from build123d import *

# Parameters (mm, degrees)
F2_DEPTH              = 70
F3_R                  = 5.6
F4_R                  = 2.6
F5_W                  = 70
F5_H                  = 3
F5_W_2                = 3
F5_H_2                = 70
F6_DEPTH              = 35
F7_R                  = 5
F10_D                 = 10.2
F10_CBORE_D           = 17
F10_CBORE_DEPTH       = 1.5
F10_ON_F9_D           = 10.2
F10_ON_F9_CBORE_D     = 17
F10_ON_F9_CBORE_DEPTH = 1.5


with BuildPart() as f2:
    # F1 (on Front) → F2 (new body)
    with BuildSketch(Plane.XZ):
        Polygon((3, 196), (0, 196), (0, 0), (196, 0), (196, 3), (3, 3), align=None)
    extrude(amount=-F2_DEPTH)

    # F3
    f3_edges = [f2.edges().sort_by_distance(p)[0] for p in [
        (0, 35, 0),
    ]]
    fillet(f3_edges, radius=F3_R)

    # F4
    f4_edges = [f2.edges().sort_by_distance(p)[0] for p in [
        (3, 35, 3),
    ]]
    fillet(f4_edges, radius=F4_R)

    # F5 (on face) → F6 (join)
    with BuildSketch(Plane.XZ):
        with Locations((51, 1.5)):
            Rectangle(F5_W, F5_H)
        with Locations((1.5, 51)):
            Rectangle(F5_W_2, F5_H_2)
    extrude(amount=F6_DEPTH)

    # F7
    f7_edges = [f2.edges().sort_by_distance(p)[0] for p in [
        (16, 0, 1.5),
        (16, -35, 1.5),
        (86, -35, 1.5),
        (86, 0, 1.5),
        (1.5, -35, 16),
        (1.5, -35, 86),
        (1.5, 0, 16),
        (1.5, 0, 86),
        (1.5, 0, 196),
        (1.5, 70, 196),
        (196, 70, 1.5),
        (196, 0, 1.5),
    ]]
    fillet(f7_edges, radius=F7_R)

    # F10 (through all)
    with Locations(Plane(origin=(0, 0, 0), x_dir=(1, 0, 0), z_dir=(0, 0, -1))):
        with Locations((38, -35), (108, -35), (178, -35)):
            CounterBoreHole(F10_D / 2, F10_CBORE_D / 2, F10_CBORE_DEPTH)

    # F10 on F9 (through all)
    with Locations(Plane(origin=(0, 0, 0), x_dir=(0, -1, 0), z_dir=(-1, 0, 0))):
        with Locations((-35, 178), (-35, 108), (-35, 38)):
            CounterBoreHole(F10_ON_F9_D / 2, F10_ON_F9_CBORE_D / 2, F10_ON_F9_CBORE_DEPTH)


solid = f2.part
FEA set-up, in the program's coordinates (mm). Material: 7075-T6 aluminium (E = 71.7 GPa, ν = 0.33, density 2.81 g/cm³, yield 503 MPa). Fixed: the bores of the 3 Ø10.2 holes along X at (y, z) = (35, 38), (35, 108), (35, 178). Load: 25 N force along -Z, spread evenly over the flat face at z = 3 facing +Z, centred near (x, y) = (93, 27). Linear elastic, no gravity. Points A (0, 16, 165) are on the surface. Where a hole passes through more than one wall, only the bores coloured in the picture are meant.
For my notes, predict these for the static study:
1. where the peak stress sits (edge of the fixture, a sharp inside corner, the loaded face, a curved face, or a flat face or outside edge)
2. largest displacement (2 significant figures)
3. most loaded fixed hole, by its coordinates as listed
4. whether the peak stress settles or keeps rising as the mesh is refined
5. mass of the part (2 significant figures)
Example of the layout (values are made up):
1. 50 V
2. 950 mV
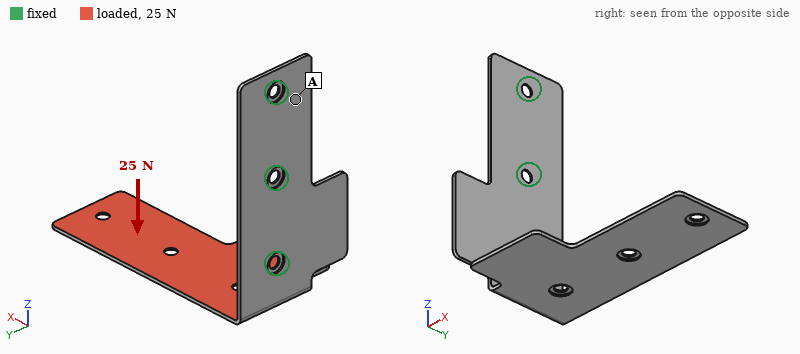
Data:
1. edge of the fixture
2. 3.0 mm
3. (35, 38)
4. keeps rising
5. 260 g
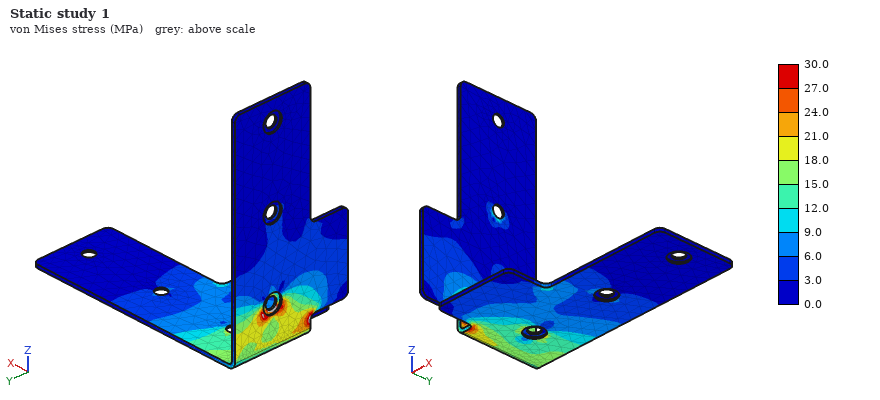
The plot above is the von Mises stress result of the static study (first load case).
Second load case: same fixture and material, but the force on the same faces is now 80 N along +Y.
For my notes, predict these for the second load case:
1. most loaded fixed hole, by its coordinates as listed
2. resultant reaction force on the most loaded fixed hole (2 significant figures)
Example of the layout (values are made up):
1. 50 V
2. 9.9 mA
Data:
1. (35, 38)
2. 180 N
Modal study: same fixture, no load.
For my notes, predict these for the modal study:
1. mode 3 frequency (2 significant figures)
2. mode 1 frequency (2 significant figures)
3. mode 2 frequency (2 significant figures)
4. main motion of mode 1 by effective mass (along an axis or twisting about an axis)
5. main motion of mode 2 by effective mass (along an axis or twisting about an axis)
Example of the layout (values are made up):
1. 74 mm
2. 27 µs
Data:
1. 270 Hz
2. 51 Hz
3. 86 Hz
4. along Z
5. along Y
